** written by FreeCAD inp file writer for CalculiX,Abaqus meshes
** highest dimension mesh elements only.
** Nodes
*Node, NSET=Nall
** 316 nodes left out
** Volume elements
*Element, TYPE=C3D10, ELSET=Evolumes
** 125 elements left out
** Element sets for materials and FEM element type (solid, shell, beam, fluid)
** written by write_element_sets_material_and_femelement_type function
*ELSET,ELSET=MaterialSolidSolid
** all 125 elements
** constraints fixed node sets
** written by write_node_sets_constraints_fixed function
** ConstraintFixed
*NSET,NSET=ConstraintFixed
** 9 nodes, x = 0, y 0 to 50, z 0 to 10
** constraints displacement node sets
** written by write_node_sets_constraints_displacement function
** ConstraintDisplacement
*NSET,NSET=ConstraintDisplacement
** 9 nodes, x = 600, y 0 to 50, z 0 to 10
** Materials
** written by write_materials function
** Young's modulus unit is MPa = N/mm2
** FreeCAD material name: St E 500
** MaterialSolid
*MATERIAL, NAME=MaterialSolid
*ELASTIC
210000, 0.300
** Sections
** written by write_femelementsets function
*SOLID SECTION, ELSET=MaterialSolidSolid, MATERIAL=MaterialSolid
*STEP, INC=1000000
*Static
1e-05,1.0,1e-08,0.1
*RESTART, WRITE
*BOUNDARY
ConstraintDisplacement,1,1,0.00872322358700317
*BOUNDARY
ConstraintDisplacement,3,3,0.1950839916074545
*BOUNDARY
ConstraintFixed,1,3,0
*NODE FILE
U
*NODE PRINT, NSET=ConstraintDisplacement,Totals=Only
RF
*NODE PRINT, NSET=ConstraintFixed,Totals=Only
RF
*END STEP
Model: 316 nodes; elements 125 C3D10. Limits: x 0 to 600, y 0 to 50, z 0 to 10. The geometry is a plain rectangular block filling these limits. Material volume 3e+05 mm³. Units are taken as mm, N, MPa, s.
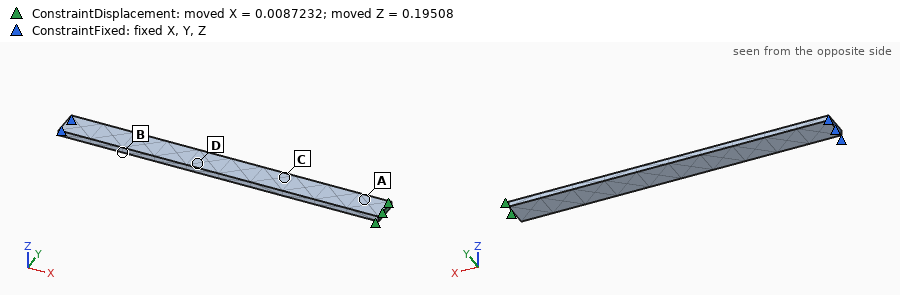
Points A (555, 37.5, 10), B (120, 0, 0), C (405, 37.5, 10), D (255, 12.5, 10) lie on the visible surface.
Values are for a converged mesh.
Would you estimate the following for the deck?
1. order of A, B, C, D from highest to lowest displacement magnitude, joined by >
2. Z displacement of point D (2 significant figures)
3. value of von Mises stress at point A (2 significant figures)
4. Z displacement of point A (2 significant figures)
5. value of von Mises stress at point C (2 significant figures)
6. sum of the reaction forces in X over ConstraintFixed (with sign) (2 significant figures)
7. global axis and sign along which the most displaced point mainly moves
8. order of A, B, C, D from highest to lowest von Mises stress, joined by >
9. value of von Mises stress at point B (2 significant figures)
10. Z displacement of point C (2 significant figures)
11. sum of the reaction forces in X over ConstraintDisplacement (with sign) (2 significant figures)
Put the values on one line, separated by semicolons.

A > C > D > B; 0.076 mm; 6.0 MPa; 0.19 mm; 4.3 MPa; -1500 N; +Z; A > B > C > D; 5.2 MPa; 0.15 mm; 1500 N
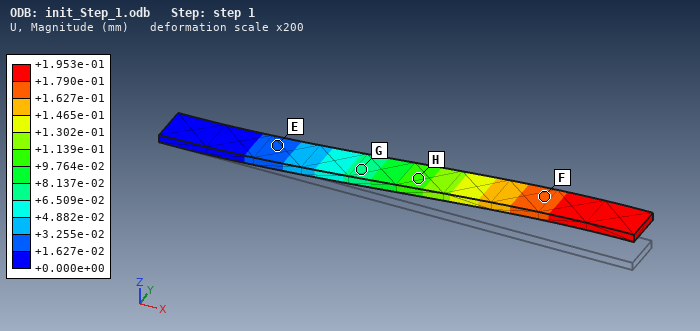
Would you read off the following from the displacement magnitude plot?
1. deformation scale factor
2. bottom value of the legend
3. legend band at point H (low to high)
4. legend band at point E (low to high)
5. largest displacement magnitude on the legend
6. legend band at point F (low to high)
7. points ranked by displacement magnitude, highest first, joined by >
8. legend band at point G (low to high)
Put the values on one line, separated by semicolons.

200; +0.000e+00 mm; +9.764e-02 to +1.139e-01 mm; +1.627e-02 to +3.255e-02 mm; +1.953e-01 mm; +1.627e-01 to +1.790e-01 mm; F > H > G > E; +6.509e-02 to +8.137e-02 mm
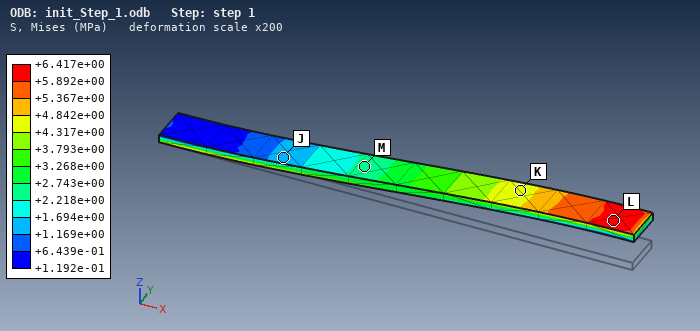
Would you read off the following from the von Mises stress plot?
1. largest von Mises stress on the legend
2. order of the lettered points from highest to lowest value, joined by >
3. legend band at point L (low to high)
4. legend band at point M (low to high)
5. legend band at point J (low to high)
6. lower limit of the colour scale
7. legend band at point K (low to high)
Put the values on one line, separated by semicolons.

+6.417e+00 MPa; L > K > M > J; +5.892e+00 to +6.417e+00 MPa; +2.218e+00 to +2.743e+00 MPa; +1.169e+00 to +1.694e+00 MPa; +1.192e-01 MPa; +4.317e+00 to +4.842e+00 MPa
